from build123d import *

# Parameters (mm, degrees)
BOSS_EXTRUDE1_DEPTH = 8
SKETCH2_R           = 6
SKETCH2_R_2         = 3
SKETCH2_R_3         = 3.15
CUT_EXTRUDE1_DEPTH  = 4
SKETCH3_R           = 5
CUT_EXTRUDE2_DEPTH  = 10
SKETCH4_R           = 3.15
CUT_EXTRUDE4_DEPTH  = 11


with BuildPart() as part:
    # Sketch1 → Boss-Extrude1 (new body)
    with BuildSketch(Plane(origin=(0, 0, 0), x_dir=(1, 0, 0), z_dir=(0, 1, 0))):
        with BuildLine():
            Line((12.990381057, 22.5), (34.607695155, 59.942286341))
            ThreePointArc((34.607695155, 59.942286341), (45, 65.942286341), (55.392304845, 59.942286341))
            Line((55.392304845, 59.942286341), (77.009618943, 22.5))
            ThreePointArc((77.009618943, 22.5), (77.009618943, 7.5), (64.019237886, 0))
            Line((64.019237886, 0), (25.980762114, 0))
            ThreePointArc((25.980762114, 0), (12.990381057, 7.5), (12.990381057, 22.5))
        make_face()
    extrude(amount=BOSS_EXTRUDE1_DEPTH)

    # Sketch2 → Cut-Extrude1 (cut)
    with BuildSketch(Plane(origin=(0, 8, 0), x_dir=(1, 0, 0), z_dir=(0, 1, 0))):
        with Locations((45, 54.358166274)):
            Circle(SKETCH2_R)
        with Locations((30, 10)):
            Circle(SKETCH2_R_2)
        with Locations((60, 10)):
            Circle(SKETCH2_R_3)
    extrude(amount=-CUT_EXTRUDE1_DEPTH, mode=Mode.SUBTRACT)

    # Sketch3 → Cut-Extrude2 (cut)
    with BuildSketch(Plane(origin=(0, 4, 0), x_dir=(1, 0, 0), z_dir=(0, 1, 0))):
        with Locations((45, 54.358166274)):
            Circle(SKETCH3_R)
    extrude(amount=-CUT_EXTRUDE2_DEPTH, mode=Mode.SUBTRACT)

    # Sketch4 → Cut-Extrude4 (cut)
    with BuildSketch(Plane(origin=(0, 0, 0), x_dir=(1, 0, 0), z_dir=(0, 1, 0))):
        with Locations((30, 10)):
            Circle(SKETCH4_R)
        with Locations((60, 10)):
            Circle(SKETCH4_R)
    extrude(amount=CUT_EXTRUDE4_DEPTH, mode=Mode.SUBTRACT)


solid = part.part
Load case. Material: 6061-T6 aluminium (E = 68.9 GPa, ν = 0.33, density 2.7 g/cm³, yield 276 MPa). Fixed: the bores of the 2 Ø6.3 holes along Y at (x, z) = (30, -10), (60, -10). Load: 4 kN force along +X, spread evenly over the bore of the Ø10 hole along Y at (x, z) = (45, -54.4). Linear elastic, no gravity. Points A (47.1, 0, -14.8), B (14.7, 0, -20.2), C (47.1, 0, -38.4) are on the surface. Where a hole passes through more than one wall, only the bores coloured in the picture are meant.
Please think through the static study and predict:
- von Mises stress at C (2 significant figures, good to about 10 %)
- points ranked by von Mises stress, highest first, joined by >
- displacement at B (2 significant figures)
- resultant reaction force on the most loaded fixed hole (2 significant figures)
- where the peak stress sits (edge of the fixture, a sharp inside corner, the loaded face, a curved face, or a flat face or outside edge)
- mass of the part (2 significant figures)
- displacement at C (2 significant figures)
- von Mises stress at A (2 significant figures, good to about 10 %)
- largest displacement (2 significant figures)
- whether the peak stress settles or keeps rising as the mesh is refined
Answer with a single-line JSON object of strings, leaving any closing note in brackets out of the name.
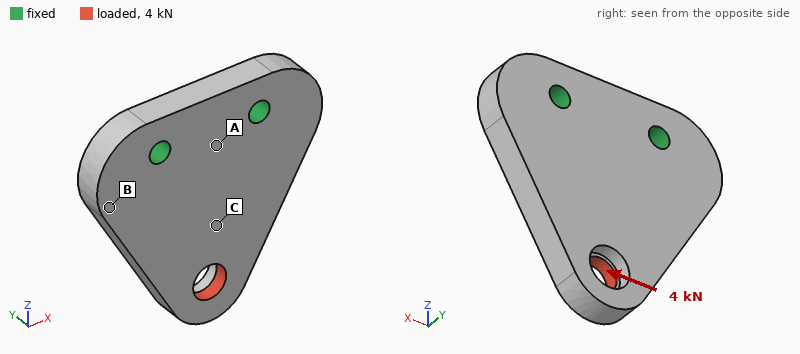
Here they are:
{"von Mises stress at C": "40 MPa", "points ranked by von Mises stress, highest first, joined by >": "C > A > B", "displacement at B": "16 µm", "resultant reaction force on the most loaded fixed hole": "5.4 kN", "where the peak stress sits": "edge of the fixture", "mass of the part": "64 g", "displacement at C": "26 µm", "von Mises stress at A": "22 MPa", "largest displacement": "67 µm", "whether the peak stress settles or keeps rising as the mesh is refined": "keeps rising"}
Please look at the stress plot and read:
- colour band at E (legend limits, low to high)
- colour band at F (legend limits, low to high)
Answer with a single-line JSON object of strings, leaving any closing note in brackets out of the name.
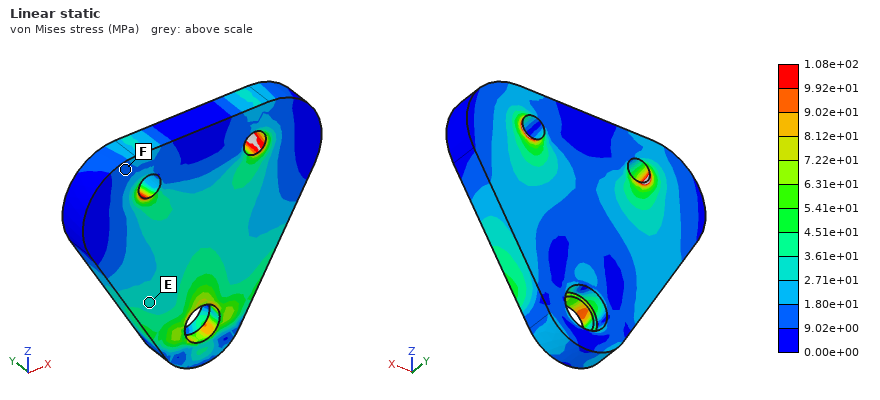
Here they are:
{"colour band at E": "2.71e+01 to 3.61e+01 MPa", "colour band at F": "9.02e+00 to 1.80e+01 MPa"}
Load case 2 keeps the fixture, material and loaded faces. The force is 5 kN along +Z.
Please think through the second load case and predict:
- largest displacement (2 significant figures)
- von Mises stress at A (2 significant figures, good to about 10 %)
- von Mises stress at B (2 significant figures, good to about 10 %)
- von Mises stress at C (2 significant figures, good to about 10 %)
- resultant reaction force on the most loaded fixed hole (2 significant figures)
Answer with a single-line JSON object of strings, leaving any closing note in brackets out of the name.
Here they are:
{"largest displacement": "0.12 mm", "von Mises stress at A": "17 MPa", "von Mises stress at B": "10 MPa", "von Mises stress at C": "41 MPa", "resultant reaction force on the most loaded fixed hole": "2.5 kN"}
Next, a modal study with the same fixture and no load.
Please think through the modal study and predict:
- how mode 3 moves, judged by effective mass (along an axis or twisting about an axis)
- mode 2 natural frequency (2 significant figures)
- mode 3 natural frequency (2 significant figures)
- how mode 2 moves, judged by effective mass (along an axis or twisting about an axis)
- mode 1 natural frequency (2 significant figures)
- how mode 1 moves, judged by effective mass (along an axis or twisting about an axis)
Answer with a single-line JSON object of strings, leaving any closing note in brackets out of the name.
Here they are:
{"how mode 3 moves, judged by effective mass": "along X", "mode 2 natural frequency": "9000 Hz", "mode 3 natural frequency": "12 kHz", "how mode 2 moves, judged by effective mass": "twisting about Z", "mode 1 natural frequency": "3200 Hz", "how mode 1 moves, judged by effective mass": "along Y"}
